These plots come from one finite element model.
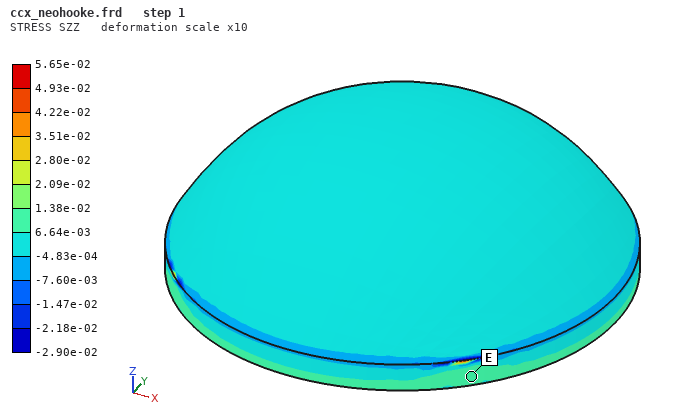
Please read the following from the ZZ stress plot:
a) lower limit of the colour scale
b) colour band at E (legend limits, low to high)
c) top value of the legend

-2.90e-02
6.64e-03 to 1.38e-02
5.65e-02
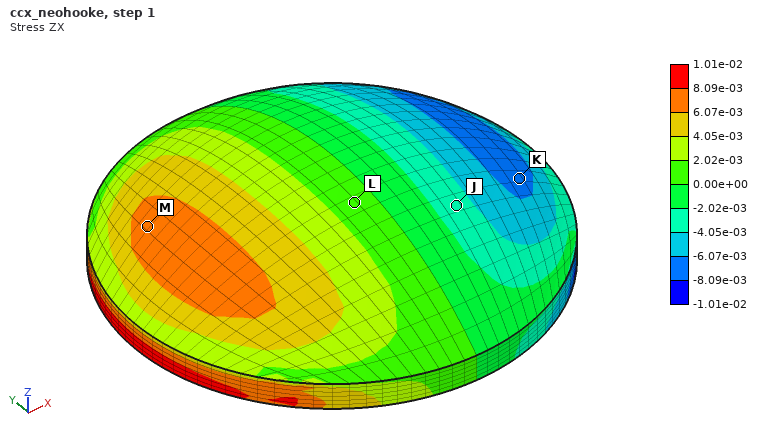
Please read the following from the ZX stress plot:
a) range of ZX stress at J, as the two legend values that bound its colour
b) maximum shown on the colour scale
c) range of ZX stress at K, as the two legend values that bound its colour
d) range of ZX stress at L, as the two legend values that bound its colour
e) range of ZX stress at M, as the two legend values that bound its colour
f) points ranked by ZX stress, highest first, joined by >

-4.05e-03 to -2.02e-03
1.01e-02
-8.09e-03 to -6.07e-03
0.00e+00 to 2.02e-03
6.07e-03 to 8.09e-03
M > L > J > K
